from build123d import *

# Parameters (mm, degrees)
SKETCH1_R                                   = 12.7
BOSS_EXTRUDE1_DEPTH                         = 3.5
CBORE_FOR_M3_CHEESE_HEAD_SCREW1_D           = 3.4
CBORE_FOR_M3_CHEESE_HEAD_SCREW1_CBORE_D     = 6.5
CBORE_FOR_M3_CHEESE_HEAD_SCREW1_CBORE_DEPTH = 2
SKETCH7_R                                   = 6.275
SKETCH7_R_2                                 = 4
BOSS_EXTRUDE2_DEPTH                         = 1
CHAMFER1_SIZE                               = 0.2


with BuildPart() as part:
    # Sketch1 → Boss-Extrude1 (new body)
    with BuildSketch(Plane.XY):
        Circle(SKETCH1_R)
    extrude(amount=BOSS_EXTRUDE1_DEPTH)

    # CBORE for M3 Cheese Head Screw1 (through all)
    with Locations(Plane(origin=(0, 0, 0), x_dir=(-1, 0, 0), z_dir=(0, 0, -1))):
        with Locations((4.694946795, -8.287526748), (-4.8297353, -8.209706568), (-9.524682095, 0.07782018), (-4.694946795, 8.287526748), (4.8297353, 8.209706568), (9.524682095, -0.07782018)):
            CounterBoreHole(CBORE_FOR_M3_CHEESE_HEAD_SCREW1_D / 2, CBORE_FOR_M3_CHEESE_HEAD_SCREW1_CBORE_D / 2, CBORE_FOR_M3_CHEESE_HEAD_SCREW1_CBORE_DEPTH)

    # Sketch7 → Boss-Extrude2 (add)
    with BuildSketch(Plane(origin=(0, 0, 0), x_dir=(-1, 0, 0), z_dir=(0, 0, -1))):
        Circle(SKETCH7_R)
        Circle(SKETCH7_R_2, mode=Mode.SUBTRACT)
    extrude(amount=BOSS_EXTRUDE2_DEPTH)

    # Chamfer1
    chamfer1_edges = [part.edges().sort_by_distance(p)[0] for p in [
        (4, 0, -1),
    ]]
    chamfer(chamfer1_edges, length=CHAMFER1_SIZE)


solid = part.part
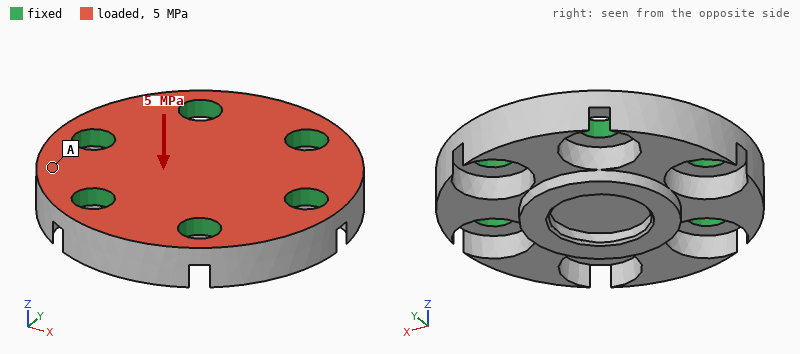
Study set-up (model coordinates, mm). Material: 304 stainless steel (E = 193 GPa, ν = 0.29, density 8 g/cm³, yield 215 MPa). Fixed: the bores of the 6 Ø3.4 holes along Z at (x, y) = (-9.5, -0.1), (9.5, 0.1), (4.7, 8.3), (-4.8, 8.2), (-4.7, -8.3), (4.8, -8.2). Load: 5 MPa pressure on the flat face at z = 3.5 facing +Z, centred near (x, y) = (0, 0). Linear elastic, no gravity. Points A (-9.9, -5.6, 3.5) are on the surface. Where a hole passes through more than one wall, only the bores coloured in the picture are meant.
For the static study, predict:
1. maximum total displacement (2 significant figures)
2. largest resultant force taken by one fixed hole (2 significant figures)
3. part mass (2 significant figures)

1.6 µm
380 N
11 g
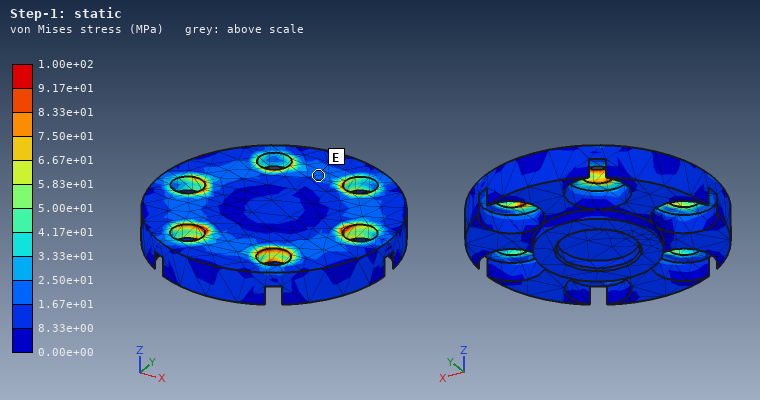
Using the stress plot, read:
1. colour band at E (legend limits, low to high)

1.67e+01 to 2.50e+01 MPa
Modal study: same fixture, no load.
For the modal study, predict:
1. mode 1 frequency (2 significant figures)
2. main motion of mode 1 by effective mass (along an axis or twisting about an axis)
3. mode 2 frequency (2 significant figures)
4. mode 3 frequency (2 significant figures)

58 kHz
along Z
75 kHz
75 kHz
